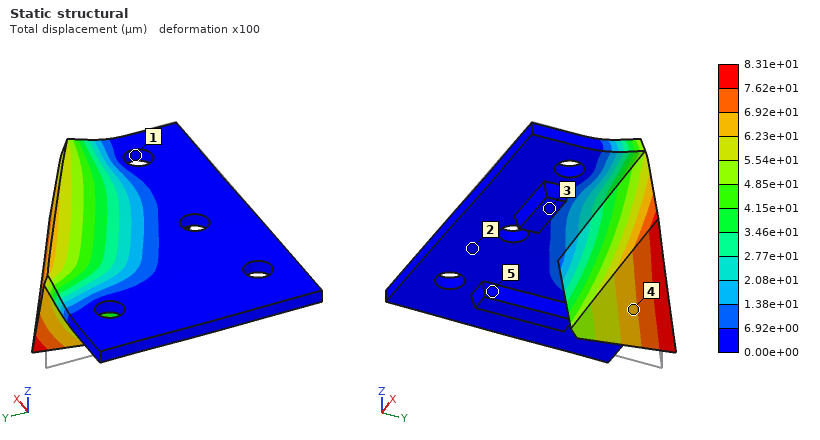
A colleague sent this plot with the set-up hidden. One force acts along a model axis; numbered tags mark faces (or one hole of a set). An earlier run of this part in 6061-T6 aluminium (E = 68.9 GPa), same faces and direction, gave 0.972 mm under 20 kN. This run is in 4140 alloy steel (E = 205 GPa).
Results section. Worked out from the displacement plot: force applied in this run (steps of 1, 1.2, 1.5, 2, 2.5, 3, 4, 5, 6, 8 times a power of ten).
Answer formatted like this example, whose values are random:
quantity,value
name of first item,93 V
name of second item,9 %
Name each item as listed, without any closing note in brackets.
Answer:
quantity,value
force applied in this run,5 kN
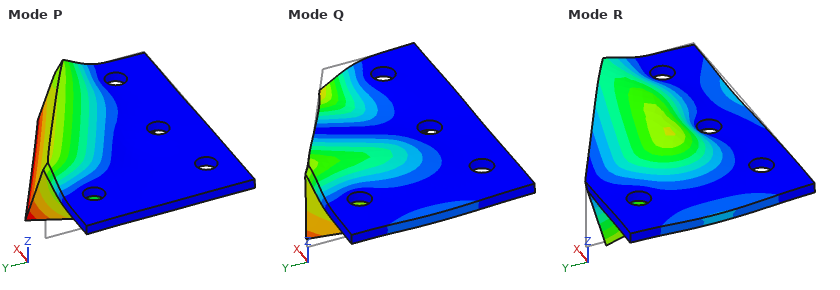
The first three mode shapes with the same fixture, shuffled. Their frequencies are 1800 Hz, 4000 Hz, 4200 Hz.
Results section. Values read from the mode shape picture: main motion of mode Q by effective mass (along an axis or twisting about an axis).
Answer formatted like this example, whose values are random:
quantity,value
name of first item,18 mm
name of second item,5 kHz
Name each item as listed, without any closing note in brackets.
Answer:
quantity,value
main motion of mode Q by effective mass,along X
